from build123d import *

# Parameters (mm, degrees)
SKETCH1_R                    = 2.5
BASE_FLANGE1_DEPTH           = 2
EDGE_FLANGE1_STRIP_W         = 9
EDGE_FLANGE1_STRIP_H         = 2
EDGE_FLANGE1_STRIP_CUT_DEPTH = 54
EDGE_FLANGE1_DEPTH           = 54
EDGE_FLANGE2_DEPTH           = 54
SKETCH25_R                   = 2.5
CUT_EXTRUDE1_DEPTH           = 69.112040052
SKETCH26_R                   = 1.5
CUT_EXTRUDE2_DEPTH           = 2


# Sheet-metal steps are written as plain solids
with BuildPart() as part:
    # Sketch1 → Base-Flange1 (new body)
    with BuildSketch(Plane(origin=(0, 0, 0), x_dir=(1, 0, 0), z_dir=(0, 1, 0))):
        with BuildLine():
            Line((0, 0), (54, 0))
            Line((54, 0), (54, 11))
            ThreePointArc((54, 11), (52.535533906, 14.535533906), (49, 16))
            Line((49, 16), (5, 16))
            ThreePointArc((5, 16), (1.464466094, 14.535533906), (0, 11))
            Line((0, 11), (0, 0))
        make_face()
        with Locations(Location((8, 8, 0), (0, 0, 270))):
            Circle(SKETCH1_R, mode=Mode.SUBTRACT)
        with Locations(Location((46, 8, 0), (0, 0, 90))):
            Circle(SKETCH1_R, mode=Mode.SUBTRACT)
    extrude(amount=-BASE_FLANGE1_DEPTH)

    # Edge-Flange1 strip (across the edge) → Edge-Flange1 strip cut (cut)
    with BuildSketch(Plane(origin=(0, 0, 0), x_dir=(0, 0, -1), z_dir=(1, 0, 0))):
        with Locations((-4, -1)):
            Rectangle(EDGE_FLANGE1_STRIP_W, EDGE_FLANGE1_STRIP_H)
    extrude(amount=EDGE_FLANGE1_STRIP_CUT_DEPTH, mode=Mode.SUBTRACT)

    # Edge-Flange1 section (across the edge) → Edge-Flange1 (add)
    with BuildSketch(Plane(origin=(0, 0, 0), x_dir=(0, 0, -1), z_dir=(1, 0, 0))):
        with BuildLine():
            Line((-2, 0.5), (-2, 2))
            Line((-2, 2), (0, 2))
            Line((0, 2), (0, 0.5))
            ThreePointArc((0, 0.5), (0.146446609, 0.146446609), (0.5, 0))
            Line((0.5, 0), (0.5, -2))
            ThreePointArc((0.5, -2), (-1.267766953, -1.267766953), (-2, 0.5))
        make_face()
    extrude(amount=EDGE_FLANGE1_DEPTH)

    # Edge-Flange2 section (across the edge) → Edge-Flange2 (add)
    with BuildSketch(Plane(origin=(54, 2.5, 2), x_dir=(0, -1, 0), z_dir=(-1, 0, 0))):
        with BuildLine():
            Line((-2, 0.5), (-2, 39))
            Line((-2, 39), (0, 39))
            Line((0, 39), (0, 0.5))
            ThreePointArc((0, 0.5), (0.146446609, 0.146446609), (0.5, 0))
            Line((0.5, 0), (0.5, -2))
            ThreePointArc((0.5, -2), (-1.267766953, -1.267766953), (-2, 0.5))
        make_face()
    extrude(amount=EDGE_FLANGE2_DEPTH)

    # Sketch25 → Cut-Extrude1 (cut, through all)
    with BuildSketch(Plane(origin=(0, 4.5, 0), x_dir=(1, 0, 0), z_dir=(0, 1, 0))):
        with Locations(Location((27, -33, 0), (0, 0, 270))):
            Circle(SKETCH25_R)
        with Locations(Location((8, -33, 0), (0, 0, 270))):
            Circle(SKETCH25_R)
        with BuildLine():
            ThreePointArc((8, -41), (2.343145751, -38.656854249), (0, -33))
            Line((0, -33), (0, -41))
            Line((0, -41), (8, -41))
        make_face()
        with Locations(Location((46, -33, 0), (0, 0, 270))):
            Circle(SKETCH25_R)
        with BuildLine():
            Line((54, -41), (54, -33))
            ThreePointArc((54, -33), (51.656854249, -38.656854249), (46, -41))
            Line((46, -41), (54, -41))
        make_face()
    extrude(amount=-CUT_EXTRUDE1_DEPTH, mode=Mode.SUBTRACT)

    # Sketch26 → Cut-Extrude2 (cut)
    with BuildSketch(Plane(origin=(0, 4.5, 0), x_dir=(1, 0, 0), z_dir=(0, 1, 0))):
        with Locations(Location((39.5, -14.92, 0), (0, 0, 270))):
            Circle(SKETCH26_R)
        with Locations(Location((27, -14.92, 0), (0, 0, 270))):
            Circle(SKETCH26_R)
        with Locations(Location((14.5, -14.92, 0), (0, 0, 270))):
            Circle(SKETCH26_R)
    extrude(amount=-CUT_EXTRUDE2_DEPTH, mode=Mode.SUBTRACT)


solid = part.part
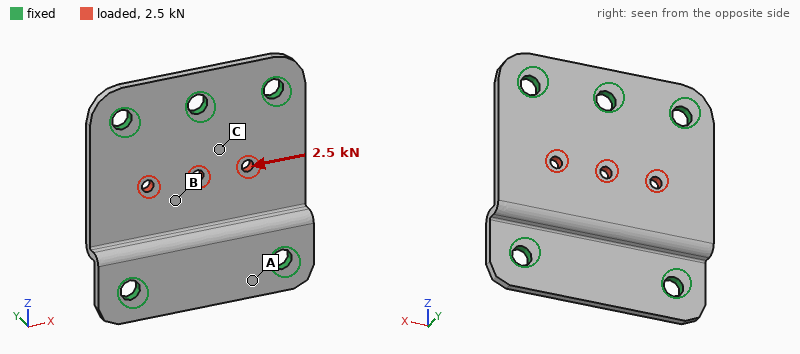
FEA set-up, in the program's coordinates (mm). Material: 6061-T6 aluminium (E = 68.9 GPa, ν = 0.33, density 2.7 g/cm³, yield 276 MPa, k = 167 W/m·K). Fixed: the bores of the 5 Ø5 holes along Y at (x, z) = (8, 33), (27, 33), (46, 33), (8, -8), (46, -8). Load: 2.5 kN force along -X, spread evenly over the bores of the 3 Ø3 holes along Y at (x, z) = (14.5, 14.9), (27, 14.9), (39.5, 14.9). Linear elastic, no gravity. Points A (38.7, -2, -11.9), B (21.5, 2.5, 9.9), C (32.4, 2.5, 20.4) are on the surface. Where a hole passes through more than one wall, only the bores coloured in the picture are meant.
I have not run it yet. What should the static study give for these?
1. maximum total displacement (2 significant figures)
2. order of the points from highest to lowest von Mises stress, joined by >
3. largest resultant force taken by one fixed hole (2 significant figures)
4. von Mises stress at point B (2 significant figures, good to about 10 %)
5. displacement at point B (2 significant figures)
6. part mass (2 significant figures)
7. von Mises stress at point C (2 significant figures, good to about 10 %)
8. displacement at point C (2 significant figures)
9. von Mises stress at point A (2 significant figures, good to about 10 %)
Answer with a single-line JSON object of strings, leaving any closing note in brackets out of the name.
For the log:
{"maximum total displacement": "17 µm", "order of the points from highest to lowest von Mises stress, joined by >": "C > B > A", "largest resultant force taken by one fixed hole": "610 N", "von Mises stress at point B": "23 MPa", "displacement at point B": "11 µm", "part mass": "17 g", "von Mises stress at point C": "34 MPa", "displacement at point C": "8.3 µm", "von Mises stress at point A": "6.6 MPa"}
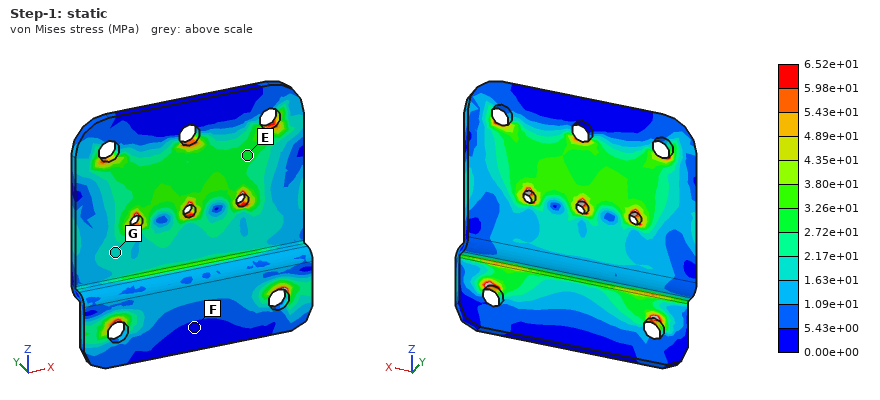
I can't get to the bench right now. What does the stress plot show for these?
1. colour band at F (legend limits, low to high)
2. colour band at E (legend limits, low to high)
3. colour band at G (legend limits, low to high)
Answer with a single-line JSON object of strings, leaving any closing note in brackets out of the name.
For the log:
{"colour band at F": "0.00e+00 to 5.43e+00 MPa", "colour band at E": "2.72e+01 to 3.26e+01 MPa", "colour band at G": "1.63e+01 to 2.17e+01 MPa"}
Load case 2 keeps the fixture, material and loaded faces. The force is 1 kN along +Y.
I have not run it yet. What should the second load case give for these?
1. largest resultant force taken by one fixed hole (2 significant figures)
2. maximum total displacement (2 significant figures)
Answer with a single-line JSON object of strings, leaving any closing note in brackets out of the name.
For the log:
{"largest resultant force taken by one fixed hole": "680 N", "maximum total displacement": "0.12 mm"}
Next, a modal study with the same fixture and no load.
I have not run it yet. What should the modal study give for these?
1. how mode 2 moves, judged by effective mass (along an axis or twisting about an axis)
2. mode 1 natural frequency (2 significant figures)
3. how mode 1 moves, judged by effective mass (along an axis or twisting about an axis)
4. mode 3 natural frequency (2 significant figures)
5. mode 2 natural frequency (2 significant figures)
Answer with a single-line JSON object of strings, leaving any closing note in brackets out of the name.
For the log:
{"how mode 2 moves, judged by effective mass": "twisting about Z", "mode 1 natural frequency": "8200 Hz", "how mode 1 moves, judged by effective mass": "along Y", "mode 3 natural frequency": "10 kHz", "mode 2 natural frequency": "9600 Hz"}
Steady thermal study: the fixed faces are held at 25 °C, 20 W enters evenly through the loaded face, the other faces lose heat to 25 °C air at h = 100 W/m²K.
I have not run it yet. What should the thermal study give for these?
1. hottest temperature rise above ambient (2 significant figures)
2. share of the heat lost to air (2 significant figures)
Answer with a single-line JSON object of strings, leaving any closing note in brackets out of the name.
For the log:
{"hottest temperature rise above ambient": "15 K", "share of the heat lost to air": "15 %"}
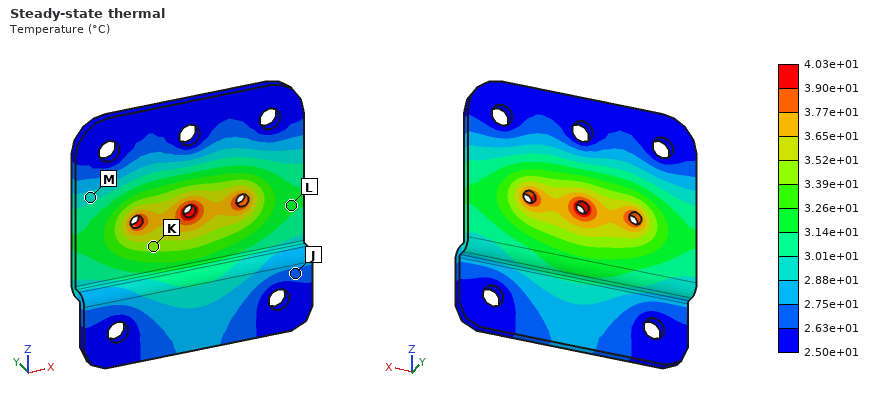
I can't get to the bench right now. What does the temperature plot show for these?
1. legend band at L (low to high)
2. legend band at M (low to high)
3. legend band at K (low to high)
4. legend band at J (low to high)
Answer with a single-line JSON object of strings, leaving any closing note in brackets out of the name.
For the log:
{"legend band at L": "3.14e+01 to 3.26e+01 °C", "legend band at M": "2.88e+01 to 3.01e+01 °C", "legend band at K": "3.39e+01 to 3.52e+01 °C", "legend band at J": "2.63e+01 to 2.75e+01 °C"}
